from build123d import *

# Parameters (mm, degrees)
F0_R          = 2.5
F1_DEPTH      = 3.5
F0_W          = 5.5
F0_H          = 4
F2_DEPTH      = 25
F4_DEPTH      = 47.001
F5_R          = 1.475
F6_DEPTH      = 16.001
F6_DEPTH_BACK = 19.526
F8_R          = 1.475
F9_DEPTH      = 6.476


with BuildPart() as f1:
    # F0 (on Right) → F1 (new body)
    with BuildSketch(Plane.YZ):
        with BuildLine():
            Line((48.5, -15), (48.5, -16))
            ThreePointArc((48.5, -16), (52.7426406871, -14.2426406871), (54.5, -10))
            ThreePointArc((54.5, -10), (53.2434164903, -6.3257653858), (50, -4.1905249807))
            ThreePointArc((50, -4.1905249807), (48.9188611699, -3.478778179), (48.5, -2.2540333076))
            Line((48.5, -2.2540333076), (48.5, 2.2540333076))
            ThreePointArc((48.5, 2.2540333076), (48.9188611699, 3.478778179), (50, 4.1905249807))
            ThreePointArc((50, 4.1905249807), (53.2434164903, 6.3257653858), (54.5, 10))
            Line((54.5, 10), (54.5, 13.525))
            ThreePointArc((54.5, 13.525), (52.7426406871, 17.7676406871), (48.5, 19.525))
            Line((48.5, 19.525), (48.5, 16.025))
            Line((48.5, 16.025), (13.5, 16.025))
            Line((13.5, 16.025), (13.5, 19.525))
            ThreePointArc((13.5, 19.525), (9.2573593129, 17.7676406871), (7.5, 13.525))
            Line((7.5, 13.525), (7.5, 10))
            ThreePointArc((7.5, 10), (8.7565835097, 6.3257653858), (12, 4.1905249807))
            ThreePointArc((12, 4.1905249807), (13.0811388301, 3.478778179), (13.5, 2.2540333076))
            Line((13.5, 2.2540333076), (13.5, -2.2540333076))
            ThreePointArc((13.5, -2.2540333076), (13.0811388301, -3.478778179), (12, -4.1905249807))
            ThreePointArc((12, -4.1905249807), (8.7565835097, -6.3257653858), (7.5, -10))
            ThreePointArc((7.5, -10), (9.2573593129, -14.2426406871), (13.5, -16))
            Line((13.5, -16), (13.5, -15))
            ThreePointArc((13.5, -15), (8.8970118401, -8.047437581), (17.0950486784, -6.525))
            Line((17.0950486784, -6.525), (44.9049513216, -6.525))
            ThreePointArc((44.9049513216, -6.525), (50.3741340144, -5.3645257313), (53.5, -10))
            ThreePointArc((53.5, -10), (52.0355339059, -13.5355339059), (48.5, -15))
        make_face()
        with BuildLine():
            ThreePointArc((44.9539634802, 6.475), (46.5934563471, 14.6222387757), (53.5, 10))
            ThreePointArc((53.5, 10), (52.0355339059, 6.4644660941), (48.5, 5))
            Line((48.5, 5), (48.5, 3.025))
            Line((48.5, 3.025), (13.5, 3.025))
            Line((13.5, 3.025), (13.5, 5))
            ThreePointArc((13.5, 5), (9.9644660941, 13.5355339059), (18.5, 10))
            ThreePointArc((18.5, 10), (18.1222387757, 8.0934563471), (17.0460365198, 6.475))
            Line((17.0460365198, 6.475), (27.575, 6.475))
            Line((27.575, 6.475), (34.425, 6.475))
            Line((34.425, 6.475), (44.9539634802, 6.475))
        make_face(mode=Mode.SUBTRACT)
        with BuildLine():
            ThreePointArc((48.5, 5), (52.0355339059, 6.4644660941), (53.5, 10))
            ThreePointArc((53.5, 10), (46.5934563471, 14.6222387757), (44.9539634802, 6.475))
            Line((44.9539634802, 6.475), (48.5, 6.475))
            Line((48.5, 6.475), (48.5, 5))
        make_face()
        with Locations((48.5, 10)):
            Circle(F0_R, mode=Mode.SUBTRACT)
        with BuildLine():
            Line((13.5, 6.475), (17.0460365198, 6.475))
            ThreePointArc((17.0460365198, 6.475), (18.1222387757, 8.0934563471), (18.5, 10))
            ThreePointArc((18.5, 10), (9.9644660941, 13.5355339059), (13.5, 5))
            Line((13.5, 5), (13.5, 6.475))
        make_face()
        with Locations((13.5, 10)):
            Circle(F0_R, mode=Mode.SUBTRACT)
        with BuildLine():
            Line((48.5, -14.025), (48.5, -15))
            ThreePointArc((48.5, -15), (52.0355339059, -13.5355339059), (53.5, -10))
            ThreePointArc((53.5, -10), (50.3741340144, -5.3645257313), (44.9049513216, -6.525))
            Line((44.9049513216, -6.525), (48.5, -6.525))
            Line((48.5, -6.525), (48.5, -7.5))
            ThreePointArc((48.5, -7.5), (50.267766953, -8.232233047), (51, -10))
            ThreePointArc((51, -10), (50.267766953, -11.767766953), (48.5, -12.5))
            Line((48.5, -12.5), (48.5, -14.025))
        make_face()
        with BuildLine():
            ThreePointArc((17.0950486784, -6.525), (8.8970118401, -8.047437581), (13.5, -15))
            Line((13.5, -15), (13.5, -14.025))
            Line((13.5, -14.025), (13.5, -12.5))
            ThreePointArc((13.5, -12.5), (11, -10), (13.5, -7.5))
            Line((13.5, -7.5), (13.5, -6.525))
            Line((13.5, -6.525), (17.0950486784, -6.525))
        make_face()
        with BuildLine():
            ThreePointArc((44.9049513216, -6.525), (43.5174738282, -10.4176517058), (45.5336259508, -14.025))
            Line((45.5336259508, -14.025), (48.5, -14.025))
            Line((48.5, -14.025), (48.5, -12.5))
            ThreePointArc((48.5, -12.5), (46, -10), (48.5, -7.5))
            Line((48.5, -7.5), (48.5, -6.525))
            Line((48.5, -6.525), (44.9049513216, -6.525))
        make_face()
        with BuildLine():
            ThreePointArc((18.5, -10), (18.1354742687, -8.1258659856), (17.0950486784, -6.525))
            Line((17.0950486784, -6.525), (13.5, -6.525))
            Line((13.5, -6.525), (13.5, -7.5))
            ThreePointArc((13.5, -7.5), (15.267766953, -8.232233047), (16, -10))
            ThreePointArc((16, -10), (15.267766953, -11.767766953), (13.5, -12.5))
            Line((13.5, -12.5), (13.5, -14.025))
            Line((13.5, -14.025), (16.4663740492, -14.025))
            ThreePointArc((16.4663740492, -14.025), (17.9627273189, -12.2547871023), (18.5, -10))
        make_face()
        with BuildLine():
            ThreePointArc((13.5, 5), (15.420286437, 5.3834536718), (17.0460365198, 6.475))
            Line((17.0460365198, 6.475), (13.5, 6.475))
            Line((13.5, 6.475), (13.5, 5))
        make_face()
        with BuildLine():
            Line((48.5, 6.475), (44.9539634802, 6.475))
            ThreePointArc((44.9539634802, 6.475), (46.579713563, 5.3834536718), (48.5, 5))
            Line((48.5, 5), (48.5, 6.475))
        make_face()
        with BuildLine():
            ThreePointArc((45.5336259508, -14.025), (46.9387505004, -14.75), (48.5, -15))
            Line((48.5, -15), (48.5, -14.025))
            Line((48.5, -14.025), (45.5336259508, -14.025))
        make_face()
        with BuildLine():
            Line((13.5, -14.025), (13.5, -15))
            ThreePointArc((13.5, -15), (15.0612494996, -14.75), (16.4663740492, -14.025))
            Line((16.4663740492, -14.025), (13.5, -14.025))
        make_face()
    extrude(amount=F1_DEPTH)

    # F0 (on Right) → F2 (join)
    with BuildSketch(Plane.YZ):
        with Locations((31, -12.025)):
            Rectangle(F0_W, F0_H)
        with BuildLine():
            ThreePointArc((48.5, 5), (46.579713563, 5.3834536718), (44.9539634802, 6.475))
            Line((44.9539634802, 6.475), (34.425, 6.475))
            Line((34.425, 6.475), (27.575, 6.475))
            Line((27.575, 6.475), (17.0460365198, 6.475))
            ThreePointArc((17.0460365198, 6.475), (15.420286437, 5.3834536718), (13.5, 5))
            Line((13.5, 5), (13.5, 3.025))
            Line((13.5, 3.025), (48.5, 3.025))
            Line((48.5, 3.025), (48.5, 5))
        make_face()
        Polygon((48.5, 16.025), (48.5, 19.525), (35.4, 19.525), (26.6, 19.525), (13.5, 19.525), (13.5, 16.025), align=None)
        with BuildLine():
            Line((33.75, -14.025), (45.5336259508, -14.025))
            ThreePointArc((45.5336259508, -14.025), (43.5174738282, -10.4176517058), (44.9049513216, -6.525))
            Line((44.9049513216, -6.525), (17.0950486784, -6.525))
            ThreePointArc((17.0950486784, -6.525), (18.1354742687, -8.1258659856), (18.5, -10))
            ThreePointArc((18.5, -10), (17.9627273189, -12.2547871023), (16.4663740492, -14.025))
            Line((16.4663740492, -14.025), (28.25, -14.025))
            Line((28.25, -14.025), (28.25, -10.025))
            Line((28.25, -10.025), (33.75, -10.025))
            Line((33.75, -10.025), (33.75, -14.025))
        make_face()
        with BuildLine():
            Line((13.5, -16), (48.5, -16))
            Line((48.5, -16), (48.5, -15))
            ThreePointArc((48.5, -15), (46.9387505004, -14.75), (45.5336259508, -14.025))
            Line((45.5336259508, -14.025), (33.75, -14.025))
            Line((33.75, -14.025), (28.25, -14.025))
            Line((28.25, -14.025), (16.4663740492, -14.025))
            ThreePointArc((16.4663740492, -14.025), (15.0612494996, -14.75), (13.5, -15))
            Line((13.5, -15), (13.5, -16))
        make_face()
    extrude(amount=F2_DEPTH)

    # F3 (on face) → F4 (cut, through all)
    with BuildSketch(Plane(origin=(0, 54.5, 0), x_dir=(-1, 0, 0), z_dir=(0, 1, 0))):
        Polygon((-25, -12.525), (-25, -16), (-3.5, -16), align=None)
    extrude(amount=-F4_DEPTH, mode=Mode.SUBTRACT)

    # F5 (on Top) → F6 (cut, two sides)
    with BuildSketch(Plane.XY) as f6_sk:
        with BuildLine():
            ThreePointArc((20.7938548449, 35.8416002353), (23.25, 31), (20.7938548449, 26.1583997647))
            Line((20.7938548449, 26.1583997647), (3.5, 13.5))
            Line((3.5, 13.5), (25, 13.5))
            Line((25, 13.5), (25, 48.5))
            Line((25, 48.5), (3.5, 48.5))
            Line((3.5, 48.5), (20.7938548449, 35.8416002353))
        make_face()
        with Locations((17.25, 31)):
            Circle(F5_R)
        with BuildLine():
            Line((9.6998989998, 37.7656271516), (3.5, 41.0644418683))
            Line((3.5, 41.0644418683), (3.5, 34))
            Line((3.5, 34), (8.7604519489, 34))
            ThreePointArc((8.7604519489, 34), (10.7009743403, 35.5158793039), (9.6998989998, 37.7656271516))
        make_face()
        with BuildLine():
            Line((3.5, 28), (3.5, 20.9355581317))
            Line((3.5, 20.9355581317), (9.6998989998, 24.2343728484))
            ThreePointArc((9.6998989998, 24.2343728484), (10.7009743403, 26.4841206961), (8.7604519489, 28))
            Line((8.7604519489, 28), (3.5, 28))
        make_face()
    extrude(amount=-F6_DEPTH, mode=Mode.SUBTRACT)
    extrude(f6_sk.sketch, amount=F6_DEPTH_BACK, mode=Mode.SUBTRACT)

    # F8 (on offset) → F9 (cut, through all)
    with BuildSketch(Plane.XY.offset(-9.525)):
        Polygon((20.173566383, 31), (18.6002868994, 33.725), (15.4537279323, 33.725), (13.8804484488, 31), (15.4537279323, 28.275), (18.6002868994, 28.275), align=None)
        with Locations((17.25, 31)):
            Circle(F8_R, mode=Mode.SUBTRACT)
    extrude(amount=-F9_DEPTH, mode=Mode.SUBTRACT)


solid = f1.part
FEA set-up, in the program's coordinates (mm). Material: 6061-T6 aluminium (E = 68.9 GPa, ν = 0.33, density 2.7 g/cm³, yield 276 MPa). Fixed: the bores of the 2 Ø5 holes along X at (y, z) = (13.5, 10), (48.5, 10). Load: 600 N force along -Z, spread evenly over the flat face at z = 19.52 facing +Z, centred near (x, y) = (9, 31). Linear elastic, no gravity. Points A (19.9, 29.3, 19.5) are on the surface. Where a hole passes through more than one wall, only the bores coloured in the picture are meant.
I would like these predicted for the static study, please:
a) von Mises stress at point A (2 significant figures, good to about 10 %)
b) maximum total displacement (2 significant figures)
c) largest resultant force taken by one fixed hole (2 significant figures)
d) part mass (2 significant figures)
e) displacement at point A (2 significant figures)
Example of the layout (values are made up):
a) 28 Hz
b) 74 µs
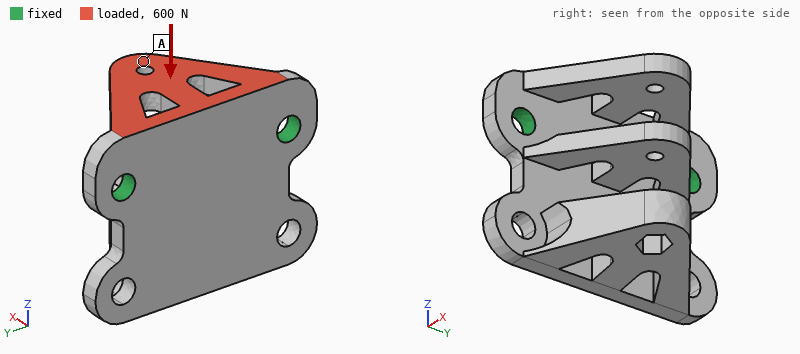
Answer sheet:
a) 11 MPa
b) 0.17 mm
c) 300 N
d) 26 g
e) 0.14 mm
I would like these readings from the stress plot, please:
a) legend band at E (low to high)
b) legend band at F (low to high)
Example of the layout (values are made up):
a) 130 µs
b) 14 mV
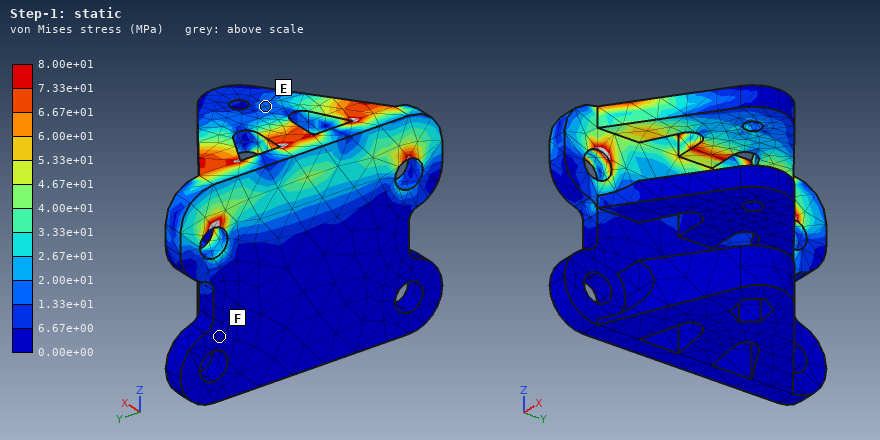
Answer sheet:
a) 1.33e+01 to 2.00e+01 MPa
b) 0.00e+00 to 6.67e+00 MPa
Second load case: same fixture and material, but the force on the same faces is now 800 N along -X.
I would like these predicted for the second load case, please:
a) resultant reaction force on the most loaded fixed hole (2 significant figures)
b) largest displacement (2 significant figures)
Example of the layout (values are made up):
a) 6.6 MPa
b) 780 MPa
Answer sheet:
a) 420 N
b) 0.11 mm
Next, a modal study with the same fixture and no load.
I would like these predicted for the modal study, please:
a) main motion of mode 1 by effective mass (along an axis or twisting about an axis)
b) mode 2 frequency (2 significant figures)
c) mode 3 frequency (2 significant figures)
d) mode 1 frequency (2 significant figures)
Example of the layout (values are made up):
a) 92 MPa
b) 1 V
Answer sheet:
a) along X
b) 5700 Hz
c) 6000 Hz
d) 2300 Hz
